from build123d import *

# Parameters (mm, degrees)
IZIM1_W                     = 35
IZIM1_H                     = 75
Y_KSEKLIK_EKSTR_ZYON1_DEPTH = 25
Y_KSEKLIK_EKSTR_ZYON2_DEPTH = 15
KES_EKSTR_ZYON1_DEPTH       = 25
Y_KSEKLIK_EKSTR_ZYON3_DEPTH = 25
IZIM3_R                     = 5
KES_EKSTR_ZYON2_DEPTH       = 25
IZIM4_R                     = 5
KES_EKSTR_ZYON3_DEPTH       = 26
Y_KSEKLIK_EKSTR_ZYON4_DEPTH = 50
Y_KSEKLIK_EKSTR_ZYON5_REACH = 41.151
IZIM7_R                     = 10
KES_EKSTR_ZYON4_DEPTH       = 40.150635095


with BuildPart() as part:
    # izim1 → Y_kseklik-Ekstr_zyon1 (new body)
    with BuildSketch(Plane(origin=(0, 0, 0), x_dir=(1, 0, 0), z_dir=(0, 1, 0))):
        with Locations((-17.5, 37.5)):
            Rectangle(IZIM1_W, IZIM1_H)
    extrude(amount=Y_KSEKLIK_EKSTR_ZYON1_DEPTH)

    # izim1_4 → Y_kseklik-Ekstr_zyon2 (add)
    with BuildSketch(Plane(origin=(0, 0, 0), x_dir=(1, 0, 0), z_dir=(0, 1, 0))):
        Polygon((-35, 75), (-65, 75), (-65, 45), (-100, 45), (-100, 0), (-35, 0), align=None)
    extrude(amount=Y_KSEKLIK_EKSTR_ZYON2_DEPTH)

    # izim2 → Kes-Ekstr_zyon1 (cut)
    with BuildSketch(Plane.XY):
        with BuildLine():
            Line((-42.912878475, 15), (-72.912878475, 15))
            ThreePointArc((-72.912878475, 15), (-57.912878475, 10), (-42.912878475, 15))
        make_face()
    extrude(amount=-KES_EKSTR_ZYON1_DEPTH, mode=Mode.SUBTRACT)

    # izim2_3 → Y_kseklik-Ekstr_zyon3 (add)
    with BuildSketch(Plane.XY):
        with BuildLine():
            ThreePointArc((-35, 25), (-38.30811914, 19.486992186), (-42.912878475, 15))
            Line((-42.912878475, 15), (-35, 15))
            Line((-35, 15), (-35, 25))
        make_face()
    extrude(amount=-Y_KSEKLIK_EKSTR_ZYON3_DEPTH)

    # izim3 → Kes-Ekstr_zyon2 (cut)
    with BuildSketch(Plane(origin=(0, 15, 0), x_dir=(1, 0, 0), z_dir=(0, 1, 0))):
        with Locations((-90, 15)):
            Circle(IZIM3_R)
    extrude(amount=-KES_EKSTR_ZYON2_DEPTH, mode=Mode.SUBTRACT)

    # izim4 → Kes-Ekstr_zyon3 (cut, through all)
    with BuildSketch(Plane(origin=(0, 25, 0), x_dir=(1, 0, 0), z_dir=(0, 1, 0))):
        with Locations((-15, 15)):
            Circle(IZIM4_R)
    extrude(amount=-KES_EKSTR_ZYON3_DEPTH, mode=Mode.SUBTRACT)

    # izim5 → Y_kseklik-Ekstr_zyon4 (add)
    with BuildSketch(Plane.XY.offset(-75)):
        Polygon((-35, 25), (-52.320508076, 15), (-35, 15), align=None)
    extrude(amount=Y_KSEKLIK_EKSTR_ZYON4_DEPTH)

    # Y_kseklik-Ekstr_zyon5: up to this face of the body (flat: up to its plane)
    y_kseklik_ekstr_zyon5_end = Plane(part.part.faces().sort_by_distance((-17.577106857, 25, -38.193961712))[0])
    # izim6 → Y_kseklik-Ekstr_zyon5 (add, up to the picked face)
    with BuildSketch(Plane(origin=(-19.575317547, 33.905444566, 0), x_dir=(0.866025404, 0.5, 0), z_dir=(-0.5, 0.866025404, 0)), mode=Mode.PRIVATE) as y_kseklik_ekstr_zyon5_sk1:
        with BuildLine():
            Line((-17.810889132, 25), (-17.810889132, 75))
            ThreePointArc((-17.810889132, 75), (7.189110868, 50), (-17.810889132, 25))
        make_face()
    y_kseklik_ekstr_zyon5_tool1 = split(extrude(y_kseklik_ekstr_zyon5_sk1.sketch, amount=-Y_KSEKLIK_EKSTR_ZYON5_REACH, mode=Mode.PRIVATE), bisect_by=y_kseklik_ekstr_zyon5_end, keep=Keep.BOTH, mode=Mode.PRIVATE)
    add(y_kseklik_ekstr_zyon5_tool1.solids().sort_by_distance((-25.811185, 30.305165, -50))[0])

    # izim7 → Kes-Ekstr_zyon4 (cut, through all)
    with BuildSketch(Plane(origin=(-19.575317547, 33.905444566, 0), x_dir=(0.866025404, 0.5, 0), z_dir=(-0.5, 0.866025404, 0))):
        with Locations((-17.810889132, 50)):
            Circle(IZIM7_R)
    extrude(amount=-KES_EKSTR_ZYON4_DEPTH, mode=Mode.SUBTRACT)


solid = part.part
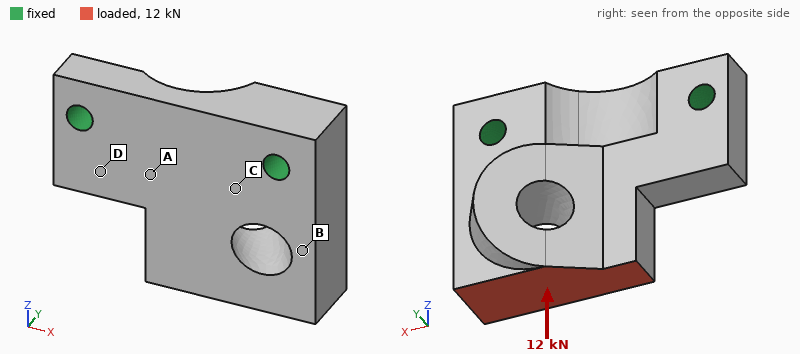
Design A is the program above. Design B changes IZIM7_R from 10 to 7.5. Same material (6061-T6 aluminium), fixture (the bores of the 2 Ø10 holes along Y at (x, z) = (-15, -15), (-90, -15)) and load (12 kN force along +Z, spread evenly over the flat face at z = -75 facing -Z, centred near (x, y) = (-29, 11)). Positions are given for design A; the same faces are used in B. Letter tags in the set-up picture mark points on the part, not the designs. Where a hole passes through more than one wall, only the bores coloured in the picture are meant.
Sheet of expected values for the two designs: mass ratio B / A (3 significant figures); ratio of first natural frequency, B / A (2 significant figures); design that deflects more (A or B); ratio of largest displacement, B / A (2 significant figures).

1.03
1.0
A
0.81
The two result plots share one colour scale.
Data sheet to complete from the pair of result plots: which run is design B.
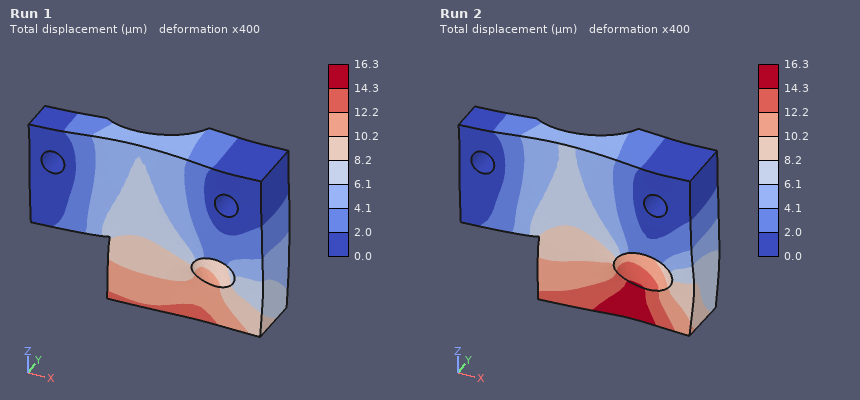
Run 1
